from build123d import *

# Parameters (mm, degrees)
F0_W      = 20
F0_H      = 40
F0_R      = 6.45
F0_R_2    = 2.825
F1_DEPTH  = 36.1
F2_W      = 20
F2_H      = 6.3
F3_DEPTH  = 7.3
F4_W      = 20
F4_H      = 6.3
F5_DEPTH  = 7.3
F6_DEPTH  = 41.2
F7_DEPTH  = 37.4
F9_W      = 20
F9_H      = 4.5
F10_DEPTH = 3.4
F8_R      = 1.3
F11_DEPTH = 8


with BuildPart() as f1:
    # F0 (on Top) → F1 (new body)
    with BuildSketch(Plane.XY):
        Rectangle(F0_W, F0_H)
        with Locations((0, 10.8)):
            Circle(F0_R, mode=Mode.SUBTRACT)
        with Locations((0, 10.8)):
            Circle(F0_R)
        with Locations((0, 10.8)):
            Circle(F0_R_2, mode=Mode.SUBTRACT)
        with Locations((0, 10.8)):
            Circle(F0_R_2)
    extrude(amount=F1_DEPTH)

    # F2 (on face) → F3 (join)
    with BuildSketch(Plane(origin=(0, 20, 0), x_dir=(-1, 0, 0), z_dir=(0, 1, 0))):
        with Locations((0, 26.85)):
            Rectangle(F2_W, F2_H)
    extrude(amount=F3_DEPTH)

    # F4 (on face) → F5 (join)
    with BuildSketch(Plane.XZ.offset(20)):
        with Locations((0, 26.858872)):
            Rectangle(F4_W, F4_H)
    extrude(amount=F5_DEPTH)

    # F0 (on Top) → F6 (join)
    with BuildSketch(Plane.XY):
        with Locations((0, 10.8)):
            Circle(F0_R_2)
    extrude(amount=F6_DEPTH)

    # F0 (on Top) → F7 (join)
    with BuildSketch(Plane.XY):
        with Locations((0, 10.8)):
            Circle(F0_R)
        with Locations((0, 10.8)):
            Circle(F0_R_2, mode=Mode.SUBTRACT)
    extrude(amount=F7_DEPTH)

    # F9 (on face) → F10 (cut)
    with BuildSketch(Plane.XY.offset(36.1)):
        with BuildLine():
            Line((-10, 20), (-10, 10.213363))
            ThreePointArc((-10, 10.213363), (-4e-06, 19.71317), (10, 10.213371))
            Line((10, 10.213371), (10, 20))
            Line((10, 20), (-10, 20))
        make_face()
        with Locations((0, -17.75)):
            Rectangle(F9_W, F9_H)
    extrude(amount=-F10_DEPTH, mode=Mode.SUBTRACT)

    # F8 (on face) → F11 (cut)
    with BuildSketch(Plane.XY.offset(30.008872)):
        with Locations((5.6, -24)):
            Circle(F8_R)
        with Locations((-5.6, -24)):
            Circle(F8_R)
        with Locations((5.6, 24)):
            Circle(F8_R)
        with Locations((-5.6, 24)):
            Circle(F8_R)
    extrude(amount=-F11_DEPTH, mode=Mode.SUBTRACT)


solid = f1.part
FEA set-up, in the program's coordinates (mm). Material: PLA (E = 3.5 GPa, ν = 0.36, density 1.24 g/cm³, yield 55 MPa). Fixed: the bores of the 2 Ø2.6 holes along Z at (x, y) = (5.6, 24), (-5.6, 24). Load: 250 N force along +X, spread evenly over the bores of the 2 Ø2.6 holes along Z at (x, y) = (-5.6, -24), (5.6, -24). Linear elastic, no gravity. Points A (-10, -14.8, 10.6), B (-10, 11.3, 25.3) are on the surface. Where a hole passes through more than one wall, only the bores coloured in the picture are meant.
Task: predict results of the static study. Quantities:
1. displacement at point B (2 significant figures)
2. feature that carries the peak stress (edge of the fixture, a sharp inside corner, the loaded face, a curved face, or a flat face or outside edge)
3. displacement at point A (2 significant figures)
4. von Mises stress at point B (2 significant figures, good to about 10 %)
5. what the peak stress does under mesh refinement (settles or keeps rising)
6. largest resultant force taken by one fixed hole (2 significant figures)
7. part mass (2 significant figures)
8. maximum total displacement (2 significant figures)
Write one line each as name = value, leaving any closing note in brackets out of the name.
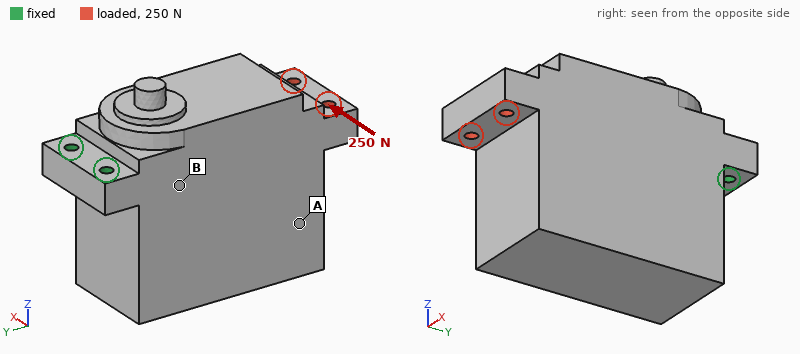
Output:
displacement at point B = 0.12 mm
feature that carries the peak stress = edge of the fixture
displacement at point A = 0.35 mm
von Mises stress at point B = 8.8 MPa
what the peak stress does under mesh refinement = keeps rising
largest resultant force taken by one fixed hole = 950 N
part mass = 38 g
maximum total displacement = 0.52 mm
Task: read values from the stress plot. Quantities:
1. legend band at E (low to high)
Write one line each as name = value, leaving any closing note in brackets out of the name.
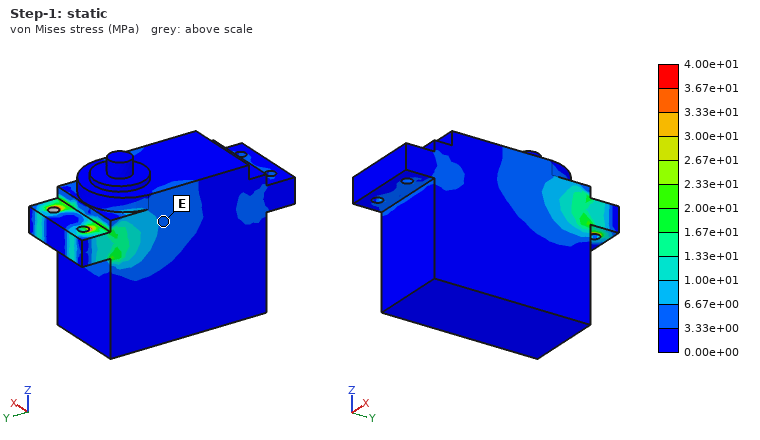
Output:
legend band at E = 3.33e+00 to 6.67e+00 MPa
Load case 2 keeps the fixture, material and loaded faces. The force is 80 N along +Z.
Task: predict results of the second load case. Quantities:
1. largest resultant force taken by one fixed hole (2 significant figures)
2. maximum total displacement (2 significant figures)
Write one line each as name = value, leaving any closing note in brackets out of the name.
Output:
largest resultant force taken by one fixed hole = 40 N
maximum total displacement = 0.82 mm
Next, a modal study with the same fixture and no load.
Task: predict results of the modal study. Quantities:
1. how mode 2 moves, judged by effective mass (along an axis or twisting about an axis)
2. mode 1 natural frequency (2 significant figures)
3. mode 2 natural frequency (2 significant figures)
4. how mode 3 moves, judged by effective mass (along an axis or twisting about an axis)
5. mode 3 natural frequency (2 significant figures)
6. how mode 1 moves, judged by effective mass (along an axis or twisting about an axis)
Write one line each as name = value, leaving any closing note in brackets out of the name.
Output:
how mode 2 moves, judged by effective mass = along X
mode 1 natural frequency = 440 Hz
mode 2 natural frequency = 1000 Hz
how mode 3 moves, judged by effective mass = twisting about Y
mode 3 natural frequency = 1800 Hz
how mode 1 moves, judged by effective mass = along Z
